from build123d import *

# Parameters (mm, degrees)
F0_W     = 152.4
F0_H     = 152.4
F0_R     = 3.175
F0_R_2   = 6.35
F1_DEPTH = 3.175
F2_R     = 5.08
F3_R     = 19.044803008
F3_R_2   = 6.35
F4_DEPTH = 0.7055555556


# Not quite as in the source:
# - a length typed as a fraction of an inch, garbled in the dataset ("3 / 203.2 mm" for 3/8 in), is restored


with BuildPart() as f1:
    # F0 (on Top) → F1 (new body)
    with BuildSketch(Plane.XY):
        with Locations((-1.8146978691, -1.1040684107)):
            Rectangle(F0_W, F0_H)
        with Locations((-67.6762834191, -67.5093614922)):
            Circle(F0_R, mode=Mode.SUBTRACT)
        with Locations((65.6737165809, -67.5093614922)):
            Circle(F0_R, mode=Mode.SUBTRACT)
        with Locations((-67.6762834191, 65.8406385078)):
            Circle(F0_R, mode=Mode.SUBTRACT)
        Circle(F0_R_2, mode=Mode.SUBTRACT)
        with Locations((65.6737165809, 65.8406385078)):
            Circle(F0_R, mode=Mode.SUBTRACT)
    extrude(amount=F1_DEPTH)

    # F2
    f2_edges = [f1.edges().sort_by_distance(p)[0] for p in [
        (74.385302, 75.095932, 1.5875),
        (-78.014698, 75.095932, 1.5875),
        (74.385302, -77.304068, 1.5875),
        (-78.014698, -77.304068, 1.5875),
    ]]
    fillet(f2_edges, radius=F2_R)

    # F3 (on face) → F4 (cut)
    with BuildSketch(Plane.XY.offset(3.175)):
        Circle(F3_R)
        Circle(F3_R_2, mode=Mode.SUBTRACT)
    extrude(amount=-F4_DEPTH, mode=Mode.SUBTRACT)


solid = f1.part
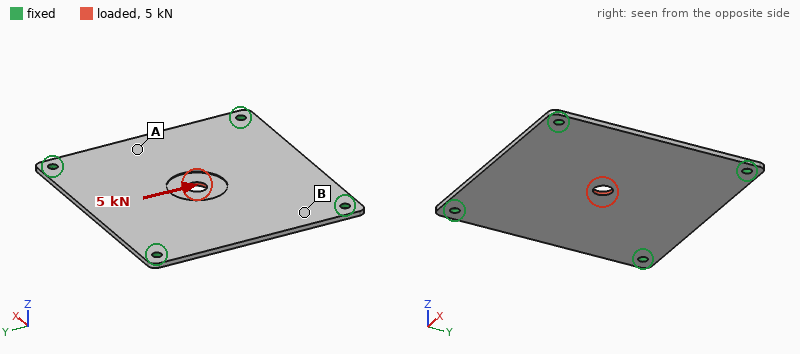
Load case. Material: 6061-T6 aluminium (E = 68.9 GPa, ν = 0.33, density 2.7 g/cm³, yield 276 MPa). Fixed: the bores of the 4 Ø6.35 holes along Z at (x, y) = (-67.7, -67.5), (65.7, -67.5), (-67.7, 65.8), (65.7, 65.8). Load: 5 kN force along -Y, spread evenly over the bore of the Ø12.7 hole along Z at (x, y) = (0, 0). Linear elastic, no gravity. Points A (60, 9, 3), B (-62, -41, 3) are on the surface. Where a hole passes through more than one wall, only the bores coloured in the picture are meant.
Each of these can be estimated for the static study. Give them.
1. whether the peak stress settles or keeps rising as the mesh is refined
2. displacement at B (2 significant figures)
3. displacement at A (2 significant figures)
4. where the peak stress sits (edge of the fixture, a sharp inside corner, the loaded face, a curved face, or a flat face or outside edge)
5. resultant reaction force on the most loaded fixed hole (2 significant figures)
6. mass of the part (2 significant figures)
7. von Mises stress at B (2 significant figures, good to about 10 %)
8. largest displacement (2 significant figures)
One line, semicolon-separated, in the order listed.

keeps rising; 6.3 µm; 7.9 µm; a sharp inside corner; 1.4 kN; 190 g; 10 MPa; 29 µm
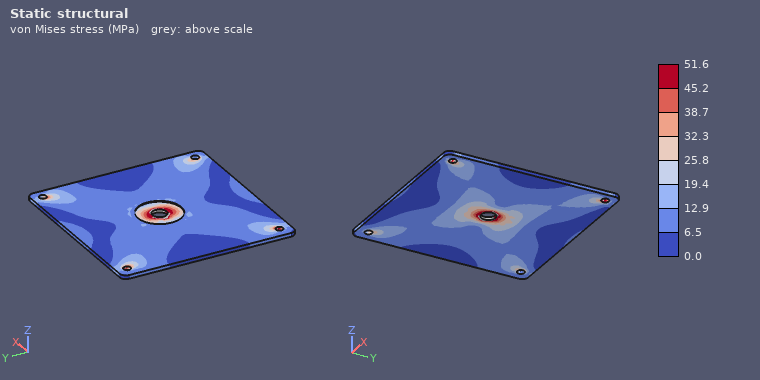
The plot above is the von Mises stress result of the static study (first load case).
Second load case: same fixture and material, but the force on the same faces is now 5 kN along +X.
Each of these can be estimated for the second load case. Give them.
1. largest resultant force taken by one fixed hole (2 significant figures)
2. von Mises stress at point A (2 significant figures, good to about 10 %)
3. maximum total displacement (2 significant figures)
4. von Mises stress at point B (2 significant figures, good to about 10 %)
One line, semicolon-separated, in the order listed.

1.4 kN; 5.8 MPa; 29 µm; 8.0 MPa
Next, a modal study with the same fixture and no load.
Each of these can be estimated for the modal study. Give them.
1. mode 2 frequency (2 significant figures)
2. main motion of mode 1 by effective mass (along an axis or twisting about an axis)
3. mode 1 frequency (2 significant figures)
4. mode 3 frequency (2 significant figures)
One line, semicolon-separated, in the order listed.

1000 Hz; along Z; 600 Hz; 1000 Hz
